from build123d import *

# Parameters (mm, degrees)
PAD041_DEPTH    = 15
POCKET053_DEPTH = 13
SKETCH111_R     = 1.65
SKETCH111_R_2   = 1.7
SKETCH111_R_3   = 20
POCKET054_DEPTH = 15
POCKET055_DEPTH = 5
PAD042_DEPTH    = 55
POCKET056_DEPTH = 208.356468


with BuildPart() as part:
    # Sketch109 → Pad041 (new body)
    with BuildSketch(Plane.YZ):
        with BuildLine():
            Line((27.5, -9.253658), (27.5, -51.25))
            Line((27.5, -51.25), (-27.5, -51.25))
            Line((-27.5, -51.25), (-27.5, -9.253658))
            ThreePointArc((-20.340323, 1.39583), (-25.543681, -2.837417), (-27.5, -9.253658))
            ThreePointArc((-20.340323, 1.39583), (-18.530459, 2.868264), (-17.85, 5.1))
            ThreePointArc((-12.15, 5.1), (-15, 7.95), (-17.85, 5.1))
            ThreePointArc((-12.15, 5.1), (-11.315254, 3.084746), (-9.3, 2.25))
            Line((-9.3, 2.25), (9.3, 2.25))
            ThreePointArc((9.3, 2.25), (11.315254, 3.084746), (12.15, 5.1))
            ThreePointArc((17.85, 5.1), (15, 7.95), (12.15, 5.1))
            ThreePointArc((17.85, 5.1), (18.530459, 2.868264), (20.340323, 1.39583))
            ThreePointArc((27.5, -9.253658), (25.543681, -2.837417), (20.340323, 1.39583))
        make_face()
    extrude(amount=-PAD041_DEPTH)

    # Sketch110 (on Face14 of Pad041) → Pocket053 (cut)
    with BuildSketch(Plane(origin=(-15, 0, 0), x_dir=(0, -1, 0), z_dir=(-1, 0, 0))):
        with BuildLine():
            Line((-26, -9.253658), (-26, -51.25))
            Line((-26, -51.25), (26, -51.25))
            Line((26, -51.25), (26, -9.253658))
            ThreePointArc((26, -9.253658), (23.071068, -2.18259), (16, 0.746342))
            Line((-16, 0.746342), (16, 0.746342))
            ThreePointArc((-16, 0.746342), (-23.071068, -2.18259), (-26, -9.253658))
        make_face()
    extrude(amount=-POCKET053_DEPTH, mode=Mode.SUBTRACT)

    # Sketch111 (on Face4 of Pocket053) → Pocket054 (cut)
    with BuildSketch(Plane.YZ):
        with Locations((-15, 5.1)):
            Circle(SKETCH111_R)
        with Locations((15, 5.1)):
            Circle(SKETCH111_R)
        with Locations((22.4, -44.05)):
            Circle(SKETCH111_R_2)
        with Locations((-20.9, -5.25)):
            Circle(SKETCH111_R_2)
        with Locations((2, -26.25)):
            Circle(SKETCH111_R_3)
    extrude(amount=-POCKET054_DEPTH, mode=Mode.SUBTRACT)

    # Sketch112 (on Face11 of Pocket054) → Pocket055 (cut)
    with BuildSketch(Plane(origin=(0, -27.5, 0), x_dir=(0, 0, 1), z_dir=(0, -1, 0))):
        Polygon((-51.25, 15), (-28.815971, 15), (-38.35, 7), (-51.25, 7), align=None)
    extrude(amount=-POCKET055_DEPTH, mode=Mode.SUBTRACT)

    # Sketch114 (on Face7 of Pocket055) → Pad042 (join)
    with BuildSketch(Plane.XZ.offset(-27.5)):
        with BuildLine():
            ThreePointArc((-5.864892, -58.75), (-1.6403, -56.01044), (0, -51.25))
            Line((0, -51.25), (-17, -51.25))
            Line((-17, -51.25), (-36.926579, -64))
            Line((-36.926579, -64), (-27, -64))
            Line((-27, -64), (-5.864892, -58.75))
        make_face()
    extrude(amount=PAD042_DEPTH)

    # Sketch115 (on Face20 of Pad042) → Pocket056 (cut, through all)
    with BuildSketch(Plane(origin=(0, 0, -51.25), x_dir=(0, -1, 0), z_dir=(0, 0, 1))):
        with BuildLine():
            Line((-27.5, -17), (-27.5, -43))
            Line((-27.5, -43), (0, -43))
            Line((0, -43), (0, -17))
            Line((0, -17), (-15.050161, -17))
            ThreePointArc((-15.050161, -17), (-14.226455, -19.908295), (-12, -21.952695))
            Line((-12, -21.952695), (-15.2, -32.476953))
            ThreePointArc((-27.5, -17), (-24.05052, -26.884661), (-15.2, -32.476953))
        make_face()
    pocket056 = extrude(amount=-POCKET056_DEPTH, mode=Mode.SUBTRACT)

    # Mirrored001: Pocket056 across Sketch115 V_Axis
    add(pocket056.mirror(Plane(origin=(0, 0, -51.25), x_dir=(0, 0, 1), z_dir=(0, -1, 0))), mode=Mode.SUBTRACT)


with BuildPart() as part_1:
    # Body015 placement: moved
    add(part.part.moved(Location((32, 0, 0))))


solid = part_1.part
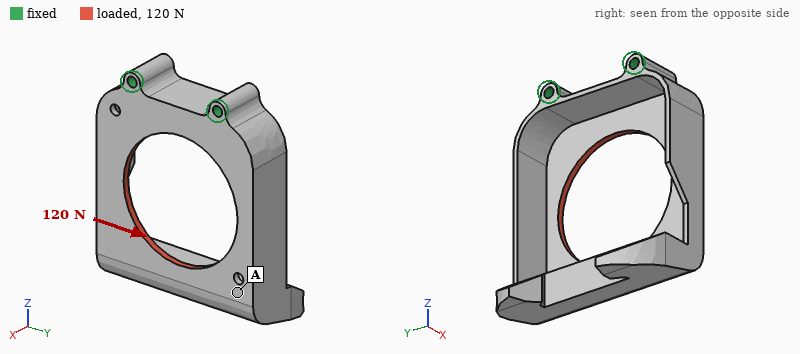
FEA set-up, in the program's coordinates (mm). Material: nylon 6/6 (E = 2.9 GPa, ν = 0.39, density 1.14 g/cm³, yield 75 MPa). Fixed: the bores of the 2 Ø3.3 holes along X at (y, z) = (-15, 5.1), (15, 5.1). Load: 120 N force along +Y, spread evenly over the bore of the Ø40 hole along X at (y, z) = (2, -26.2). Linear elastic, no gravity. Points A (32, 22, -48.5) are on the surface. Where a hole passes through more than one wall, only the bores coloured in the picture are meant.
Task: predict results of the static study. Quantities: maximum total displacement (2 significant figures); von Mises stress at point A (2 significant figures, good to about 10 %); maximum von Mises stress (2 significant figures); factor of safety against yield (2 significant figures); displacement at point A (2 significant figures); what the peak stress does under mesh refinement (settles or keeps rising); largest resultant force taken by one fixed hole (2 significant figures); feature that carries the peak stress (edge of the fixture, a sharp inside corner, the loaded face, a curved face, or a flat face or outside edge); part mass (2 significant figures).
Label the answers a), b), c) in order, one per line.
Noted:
a) 0.95 mm
b) 2.1 MPa
c) 18 MPa
d) 4.1
e) 0.62 mm
f) settles
g) 120 N
h) the loaded face
i) 19 g
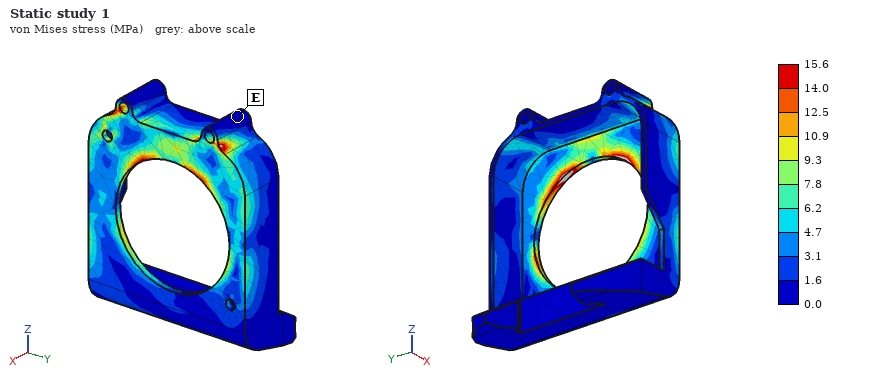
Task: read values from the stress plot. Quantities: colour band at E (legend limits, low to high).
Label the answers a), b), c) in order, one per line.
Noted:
a) 0.0 to 1.6 MPa
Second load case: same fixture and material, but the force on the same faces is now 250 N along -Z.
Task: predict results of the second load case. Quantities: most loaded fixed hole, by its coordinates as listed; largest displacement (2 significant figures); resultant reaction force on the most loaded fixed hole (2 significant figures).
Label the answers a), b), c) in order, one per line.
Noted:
a) (15, 5.1)
b) 0.48 mm
c) 140 N
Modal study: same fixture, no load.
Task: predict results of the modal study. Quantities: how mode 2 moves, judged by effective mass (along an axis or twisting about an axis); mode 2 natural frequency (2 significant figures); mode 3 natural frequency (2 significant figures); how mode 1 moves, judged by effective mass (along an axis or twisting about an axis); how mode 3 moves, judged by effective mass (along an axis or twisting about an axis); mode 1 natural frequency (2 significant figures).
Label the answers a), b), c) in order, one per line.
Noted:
a) along Y
b) 260 Hz
c) 580 Hz
d) along X
e) along Y
f) 140 Hz
